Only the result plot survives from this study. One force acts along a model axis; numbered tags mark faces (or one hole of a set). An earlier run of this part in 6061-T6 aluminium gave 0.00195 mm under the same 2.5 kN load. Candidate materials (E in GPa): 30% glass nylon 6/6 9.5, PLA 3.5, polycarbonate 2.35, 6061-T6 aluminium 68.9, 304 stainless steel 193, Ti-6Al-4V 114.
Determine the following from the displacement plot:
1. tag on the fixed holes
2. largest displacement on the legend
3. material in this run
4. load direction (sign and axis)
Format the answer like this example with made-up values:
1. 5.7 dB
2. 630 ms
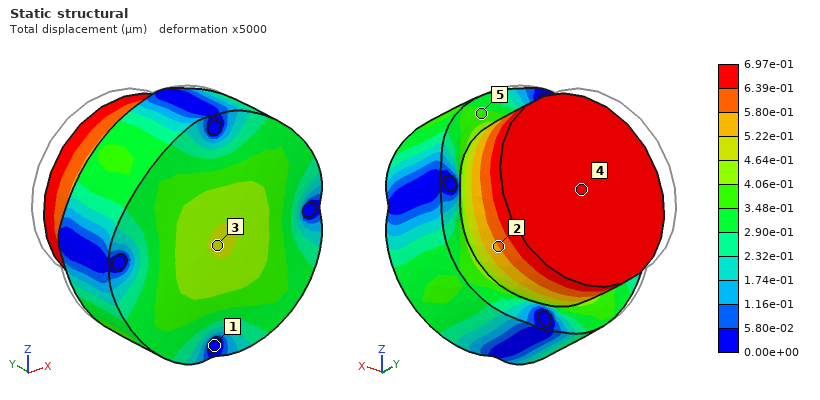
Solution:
1. 1
2. 6.97e-01 µm
3. 304 stainless steel
4. -Y
